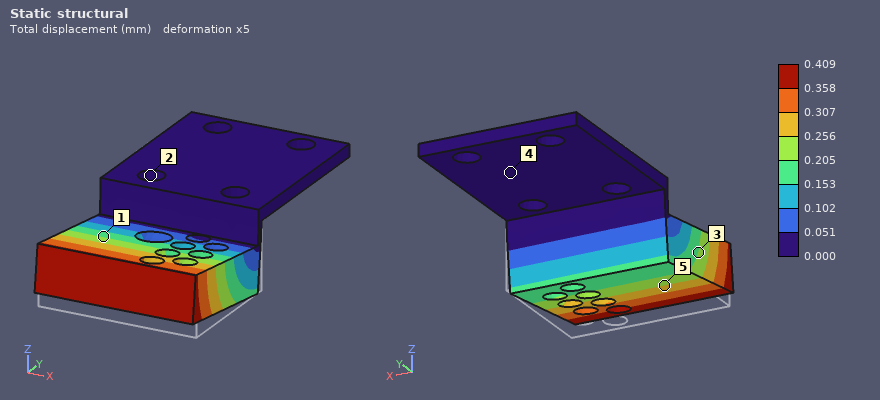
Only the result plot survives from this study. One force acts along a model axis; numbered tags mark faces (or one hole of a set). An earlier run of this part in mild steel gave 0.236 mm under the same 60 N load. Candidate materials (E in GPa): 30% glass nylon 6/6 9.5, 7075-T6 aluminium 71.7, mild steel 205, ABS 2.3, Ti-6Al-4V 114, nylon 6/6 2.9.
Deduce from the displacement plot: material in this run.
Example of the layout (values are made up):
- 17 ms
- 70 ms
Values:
- Ti-6Al-4V
